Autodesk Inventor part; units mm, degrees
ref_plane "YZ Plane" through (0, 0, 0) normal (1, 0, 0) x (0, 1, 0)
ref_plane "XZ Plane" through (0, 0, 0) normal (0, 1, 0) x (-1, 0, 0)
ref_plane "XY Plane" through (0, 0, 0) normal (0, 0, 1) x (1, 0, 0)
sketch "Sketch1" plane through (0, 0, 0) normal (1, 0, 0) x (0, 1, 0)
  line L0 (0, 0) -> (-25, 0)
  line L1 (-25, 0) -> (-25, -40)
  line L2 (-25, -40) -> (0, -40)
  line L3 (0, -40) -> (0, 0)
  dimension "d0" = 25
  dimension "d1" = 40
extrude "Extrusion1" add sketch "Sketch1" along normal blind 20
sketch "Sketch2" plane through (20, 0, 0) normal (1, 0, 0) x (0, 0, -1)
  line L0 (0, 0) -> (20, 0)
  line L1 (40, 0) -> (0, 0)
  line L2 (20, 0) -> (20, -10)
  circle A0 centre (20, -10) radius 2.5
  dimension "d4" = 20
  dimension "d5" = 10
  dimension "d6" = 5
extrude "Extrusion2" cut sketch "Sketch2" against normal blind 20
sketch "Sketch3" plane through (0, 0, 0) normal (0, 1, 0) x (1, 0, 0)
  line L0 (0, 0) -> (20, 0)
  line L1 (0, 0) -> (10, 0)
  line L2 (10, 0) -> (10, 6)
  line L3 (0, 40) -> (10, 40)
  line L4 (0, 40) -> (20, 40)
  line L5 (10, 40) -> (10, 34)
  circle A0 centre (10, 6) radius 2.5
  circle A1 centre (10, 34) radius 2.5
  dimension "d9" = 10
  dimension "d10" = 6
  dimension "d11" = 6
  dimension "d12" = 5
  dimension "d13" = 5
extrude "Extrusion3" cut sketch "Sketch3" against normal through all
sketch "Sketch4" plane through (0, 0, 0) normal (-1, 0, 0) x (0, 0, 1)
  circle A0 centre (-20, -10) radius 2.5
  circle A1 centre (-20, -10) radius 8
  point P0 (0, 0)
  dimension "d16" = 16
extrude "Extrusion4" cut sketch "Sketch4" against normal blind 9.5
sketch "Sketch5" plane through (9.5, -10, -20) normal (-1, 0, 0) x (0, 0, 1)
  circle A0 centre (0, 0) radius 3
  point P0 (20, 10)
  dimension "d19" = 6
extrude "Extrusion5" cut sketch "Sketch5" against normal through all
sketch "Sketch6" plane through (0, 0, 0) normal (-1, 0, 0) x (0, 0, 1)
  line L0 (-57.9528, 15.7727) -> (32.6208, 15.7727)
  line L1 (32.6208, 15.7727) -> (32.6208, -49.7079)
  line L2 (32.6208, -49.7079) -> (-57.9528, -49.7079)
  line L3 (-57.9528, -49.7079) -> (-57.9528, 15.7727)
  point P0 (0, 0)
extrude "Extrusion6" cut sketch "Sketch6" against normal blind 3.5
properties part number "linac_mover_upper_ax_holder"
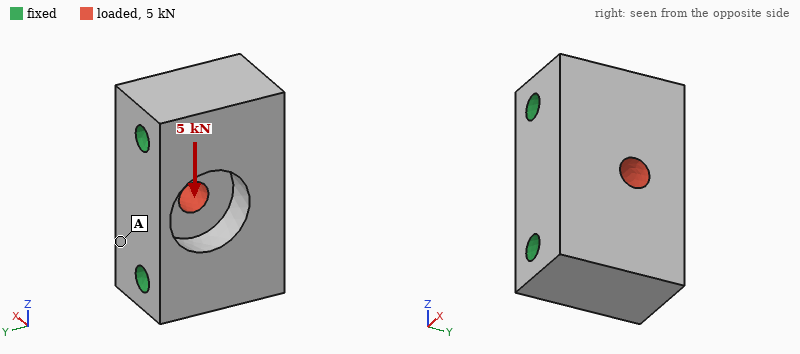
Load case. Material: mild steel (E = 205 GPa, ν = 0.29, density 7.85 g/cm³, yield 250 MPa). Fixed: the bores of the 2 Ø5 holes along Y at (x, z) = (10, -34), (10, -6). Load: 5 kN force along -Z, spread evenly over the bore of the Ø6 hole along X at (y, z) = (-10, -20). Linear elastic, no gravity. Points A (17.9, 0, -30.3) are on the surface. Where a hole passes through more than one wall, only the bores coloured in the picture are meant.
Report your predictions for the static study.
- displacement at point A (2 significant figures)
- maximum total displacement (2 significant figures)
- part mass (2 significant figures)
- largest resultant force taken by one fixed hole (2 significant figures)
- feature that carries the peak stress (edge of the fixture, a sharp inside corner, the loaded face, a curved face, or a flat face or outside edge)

0.53 µm
1.3 µm
110 g
2.6 kN
the loaded face
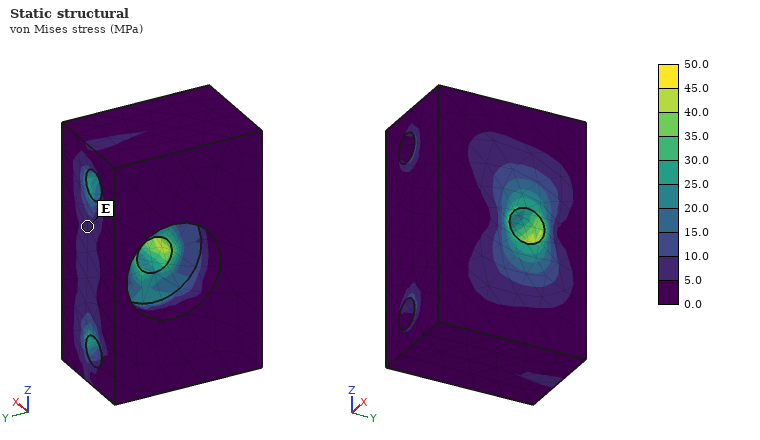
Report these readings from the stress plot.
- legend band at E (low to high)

5.0 to 10.0 MPa
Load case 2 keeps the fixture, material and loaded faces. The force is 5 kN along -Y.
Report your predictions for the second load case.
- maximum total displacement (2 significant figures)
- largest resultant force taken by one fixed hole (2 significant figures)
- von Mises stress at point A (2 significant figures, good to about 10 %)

2.4 µm
2.5 kN
5.5 MPa
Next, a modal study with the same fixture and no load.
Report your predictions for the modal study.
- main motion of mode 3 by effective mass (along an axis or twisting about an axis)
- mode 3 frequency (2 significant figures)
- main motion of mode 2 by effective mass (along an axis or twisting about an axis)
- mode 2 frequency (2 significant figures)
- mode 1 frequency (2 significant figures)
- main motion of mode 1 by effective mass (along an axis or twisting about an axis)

along Y
55 kHz
along Y
50 kHz
46 kHz
along X
